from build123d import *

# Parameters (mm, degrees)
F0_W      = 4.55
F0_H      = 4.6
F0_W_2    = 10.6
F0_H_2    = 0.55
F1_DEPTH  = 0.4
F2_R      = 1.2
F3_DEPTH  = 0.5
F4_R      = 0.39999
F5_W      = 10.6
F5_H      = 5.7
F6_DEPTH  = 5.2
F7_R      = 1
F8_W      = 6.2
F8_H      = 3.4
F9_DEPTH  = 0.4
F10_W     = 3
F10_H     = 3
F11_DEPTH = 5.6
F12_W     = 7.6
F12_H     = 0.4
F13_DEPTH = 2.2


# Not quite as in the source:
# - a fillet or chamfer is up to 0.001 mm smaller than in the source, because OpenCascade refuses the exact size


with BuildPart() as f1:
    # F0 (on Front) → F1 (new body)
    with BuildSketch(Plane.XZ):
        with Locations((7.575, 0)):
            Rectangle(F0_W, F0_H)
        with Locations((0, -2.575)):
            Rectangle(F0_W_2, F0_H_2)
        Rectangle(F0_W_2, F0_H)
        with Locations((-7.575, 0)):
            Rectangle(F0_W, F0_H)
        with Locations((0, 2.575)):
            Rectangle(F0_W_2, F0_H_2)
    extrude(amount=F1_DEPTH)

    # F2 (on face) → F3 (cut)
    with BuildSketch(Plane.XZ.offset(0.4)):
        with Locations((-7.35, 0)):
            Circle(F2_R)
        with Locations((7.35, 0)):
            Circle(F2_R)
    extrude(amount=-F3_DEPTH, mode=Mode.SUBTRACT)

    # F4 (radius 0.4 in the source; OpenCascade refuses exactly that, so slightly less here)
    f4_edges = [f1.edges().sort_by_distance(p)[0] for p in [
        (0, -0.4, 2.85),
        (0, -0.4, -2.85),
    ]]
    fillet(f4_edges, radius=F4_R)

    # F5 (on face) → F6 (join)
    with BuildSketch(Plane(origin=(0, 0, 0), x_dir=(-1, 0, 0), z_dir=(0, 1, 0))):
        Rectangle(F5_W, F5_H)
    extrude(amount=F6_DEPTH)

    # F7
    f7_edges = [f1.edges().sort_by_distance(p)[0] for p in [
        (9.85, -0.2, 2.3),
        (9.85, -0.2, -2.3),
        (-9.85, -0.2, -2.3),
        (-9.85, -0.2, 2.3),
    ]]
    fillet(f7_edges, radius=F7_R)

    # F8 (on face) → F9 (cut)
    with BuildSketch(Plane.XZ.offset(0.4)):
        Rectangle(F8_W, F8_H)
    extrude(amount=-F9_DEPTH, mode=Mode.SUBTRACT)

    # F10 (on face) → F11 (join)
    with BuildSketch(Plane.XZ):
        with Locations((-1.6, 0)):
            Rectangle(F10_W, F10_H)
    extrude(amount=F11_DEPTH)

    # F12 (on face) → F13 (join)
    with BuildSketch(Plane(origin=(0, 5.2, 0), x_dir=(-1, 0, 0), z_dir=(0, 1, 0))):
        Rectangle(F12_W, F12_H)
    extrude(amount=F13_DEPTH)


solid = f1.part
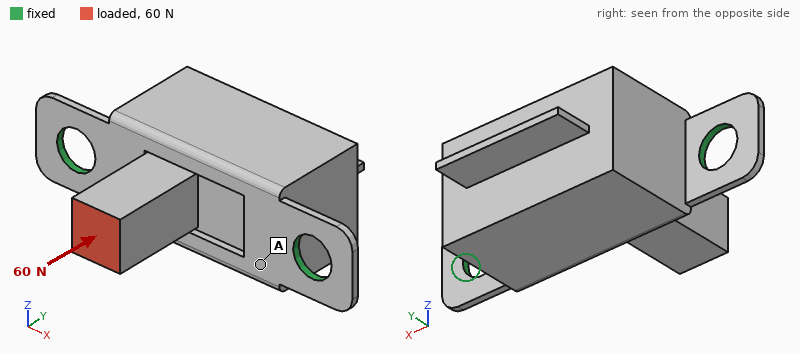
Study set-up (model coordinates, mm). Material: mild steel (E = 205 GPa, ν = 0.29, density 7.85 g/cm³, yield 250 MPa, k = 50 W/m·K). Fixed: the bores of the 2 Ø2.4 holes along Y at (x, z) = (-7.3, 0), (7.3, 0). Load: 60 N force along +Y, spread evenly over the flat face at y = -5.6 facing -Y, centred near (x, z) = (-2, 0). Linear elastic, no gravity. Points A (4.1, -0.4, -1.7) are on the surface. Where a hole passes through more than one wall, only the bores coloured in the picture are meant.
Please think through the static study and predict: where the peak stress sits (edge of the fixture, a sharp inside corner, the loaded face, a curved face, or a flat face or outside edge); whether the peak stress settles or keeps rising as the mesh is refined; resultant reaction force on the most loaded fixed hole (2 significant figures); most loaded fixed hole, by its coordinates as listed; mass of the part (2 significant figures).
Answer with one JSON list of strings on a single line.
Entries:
["edge of the fixture", "keeps rising", "43 N", "(-7.3, 0)", "3.1 g"]
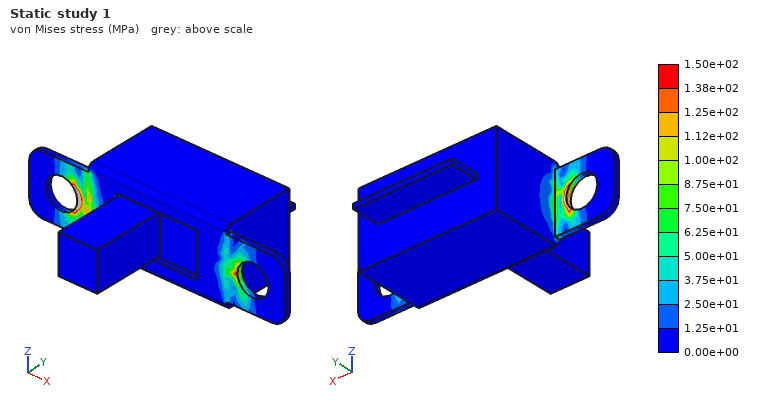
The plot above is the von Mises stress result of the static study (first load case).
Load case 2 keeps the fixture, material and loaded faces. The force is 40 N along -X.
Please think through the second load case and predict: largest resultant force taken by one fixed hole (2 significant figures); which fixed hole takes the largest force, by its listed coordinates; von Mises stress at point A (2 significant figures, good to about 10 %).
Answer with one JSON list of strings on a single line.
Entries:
["33 N", "(-7.3, 0)", "9.6 MPa"]
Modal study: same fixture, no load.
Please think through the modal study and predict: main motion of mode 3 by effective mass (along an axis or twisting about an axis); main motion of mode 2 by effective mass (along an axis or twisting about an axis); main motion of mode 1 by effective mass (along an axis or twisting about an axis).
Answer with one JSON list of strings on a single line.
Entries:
["along X", "along Y", "along Z"]
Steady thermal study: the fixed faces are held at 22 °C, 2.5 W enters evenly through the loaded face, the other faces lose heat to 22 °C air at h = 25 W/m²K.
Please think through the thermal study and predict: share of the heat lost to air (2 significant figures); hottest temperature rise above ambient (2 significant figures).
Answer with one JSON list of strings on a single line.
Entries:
["10 %", "58 K"]
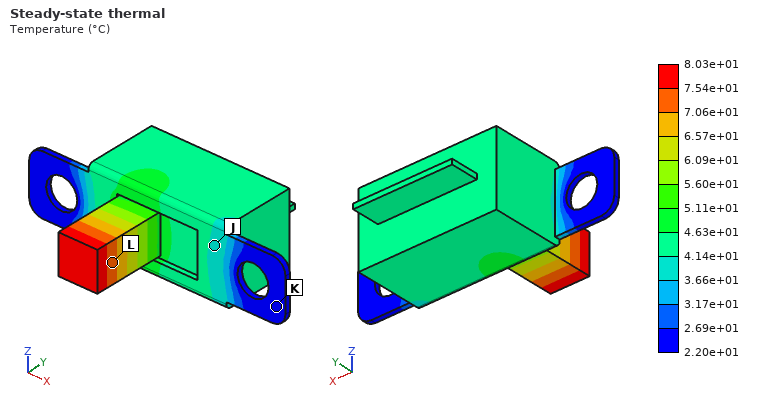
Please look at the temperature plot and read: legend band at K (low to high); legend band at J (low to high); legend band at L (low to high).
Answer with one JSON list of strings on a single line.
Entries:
["2.20e+01 to 2.69e+01 °C", "3.66e+01 to 4.14e+01 °C", "7.06e+01 to 7.54e+01 °C"]
